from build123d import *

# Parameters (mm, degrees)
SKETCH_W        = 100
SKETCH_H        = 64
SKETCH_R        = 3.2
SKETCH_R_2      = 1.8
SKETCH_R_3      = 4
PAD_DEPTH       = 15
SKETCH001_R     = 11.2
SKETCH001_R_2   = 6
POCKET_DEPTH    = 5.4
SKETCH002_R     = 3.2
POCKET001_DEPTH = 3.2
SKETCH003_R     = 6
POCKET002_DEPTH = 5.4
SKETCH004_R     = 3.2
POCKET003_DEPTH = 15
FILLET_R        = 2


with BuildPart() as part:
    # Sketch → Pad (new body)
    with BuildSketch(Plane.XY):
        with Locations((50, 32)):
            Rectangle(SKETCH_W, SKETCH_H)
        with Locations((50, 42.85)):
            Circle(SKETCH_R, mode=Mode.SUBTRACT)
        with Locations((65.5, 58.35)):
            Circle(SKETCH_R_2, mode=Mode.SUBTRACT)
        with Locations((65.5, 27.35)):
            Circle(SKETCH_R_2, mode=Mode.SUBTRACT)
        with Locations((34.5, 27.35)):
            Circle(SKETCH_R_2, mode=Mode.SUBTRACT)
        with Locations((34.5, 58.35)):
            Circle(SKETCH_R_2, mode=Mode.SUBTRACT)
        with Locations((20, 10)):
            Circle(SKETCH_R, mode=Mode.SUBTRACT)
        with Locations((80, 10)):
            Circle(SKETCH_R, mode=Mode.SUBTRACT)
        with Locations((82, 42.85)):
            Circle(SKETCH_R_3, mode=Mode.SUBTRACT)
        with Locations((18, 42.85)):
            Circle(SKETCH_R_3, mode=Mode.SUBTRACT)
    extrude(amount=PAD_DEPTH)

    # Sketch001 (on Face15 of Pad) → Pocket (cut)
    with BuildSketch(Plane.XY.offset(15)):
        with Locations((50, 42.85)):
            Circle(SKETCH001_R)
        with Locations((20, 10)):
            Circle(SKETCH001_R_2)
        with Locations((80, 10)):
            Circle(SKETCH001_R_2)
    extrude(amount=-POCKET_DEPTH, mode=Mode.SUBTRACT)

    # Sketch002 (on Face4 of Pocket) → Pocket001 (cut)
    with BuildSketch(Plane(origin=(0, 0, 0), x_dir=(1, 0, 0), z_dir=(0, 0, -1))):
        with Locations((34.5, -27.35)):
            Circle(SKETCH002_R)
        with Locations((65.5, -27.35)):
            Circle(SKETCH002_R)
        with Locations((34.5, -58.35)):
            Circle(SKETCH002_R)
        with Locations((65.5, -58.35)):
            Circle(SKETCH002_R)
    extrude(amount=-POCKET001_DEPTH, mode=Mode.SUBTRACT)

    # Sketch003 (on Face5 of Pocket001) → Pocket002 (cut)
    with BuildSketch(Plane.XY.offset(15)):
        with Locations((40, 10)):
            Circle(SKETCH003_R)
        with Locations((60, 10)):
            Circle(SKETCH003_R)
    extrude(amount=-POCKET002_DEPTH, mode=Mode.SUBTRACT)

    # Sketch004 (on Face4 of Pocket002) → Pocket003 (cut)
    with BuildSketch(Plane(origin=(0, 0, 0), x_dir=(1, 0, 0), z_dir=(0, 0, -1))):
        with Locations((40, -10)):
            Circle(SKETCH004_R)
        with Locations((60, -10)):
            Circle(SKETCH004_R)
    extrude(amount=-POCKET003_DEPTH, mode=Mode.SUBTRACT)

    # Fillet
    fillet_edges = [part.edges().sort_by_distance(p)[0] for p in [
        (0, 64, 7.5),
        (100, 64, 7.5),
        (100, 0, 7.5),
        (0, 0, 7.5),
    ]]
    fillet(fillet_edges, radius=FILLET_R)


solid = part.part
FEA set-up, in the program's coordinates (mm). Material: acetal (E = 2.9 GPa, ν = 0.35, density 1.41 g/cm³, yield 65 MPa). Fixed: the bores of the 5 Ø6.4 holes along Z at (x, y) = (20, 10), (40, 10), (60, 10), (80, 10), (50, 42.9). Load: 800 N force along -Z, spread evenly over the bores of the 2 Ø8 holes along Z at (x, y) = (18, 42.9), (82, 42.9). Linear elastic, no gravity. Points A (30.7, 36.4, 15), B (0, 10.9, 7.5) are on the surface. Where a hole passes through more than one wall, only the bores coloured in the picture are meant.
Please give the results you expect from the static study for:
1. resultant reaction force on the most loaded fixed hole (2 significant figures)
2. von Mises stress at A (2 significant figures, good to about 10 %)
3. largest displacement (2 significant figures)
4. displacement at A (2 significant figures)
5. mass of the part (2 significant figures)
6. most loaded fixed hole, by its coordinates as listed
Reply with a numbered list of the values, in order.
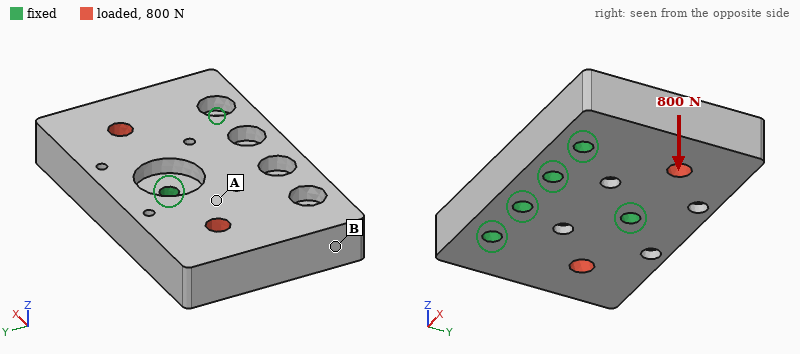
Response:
1. 540 N
2. 2.8 MPa
3. 0.19 mm
4. 0.048 mm
5. 120 g
6. (50, 42.9)
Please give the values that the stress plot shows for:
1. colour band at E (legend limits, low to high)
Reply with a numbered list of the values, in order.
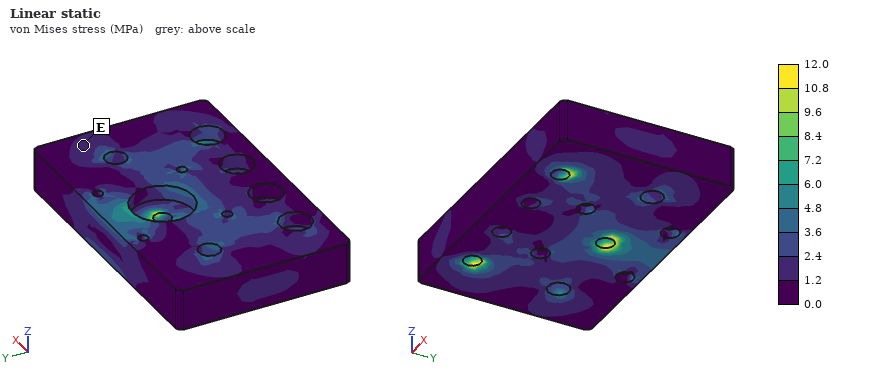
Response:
1. 1.2 to 2.4 MPa
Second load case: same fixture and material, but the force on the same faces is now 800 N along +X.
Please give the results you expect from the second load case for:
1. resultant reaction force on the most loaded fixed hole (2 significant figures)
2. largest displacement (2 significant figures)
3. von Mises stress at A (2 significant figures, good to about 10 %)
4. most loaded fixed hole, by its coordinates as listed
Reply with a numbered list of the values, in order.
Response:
1. 540 N
2. 23 µm
3. 1.0 MPa
4. (50, 42.9)
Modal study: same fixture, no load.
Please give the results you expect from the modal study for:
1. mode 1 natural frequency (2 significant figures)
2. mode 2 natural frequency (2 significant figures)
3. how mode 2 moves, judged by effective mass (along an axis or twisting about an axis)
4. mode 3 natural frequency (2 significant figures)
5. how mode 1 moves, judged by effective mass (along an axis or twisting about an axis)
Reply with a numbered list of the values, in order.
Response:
1. 1400 Hz
2. 1600 Hz
3. along Z
4. 3700 Hz
5. twisting about Y
